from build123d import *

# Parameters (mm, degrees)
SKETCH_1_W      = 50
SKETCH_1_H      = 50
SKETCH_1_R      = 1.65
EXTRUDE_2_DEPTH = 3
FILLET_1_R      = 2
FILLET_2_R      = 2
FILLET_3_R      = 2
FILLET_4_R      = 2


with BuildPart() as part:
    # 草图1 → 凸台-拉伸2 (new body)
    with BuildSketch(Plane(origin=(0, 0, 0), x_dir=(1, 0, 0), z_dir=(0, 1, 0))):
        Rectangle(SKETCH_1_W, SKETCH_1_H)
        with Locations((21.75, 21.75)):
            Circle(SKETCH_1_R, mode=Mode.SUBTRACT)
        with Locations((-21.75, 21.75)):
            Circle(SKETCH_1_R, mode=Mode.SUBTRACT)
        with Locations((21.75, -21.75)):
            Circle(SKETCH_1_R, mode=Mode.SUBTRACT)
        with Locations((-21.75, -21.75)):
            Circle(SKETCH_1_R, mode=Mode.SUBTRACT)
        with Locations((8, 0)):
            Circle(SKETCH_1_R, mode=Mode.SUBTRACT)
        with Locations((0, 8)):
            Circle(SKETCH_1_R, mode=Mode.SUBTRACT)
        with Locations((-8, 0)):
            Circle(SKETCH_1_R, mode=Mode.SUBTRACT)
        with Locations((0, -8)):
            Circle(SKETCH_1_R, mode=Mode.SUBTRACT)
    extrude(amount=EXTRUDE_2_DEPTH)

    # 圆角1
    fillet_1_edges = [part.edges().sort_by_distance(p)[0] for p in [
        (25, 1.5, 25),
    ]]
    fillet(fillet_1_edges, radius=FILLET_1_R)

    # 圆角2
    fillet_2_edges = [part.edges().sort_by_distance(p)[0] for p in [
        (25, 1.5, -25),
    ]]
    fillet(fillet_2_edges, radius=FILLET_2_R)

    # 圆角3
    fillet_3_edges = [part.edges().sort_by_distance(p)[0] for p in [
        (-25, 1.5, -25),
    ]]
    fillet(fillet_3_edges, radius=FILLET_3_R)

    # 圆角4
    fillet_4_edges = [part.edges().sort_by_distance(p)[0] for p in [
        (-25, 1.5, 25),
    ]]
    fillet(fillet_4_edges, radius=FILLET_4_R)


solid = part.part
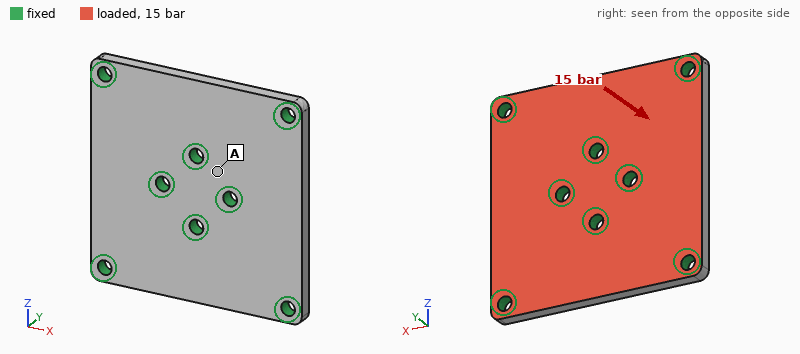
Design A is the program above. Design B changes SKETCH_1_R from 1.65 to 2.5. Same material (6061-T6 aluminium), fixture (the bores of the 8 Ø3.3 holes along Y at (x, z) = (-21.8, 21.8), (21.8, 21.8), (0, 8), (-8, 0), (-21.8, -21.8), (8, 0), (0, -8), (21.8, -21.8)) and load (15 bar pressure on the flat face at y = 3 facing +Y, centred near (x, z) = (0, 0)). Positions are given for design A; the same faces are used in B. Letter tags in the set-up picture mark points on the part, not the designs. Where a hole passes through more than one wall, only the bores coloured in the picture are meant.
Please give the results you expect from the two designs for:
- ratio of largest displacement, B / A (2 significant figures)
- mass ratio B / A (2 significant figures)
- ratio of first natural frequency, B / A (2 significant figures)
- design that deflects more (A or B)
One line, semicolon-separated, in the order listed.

0.82; 0.96; 1.1; A
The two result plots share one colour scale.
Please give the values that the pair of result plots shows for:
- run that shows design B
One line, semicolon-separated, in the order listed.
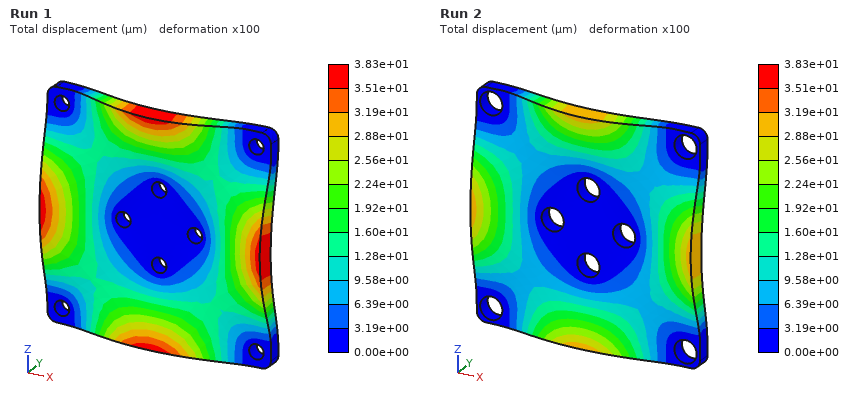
Run 2
